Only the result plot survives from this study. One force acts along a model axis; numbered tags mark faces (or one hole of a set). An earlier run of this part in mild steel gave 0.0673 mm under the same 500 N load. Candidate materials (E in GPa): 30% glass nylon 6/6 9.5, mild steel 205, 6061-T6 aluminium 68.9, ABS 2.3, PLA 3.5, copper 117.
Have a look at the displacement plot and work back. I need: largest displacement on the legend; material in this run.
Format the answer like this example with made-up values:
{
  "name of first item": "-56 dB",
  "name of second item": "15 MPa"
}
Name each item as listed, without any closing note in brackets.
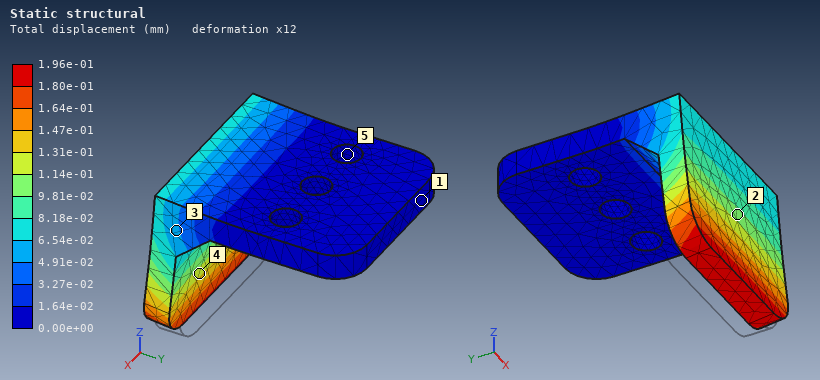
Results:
{
  "largest displacement on the legend": "1.96e-01 mm",
  "material in this run": "6061-T6 aluminium"
}
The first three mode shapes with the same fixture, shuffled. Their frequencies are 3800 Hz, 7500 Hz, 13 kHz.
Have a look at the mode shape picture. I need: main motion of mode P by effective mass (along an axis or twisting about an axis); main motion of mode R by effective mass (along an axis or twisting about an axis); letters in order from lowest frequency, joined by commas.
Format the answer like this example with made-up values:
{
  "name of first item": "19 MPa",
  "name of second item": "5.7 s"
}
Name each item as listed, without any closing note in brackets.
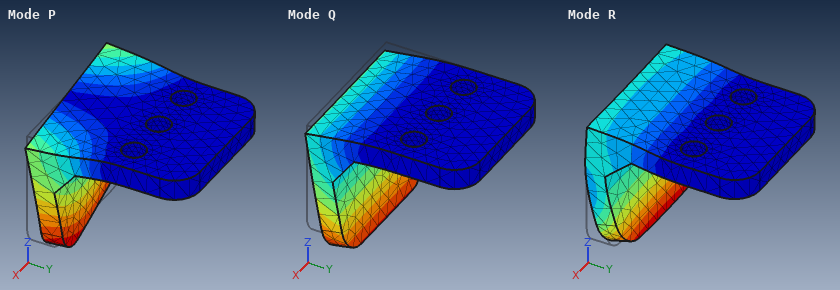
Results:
{
  "main motion of mode P by effective mass": "along X",
  "main motion of mode R by effective mass": "along Z",
  "letters in order from lowest frequency, joined by commas": "Q, P, R"
}
